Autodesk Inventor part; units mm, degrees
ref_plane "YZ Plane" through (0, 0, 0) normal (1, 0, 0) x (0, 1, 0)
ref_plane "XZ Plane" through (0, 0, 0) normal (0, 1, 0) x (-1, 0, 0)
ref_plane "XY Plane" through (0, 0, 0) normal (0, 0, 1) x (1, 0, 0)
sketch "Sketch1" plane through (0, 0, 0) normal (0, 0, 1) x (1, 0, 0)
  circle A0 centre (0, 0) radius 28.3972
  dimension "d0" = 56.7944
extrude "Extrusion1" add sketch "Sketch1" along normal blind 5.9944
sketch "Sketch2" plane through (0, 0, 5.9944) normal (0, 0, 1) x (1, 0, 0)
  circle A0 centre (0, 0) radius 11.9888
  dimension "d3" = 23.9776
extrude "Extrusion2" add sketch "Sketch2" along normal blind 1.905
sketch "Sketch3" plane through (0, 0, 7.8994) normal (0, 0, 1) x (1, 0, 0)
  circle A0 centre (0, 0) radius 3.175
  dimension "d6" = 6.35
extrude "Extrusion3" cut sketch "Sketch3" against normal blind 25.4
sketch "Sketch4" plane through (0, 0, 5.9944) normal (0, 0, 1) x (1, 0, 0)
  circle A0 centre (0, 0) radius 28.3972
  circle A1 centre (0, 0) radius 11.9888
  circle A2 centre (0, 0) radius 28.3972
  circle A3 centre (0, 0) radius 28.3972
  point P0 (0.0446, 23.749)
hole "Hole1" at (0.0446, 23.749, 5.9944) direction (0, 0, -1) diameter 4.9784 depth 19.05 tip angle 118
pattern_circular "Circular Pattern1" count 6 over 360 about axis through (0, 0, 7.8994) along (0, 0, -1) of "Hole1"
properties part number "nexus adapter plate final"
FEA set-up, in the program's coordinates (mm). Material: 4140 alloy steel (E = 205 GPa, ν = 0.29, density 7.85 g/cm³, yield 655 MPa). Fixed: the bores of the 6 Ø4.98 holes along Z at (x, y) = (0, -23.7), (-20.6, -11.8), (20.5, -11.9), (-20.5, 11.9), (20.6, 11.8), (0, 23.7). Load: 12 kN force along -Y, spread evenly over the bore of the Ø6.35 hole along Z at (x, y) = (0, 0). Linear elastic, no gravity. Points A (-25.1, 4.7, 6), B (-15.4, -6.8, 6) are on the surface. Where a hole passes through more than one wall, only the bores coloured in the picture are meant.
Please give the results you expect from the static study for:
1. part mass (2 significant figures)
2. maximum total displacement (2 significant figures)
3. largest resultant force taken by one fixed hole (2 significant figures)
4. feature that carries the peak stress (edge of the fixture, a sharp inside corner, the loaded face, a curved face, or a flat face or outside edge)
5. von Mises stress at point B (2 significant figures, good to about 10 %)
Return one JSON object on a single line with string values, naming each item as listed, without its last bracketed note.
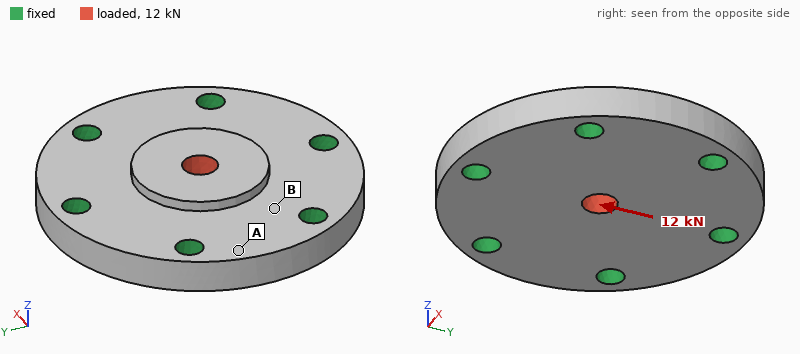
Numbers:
{"part mass": "120 g", "maximum total displacement": "5.2 µm", "largest resultant force taken by one fixed hole": "3.1 kN", "feature that carries the peak stress": "the loaded face", "von Mises stress at point B": "28 MPa"}
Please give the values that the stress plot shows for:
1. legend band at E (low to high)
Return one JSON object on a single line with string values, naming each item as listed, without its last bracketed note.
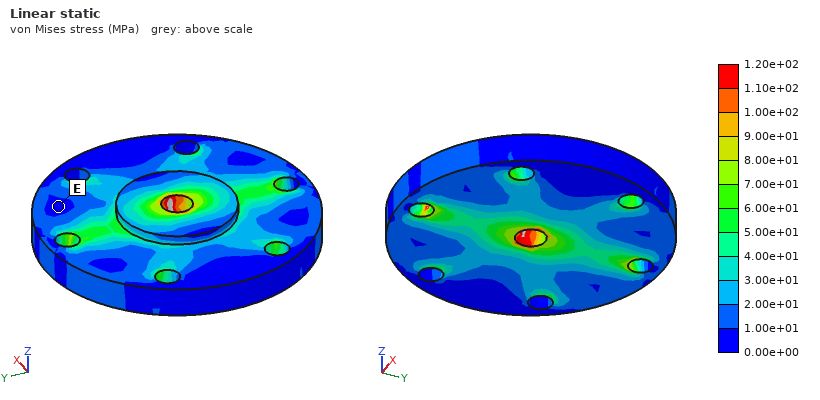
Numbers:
{"legend band at E": "0.00e+00 to 1.00e+01 MPa"}
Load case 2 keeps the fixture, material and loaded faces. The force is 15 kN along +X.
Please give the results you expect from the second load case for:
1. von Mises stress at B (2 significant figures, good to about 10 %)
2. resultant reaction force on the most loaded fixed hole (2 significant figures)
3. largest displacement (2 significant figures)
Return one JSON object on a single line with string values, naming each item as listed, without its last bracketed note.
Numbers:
{"von Mises stress at B": "57 MPa", "resultant reaction force on the most loaded fixed hole": "3.4 kN", "largest displacement": "6.6 µm"}
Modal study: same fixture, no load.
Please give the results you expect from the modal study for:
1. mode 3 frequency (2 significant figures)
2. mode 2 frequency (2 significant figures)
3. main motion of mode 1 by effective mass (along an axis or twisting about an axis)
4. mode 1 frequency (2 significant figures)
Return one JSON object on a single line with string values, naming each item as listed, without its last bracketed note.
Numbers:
{"mode 3 frequency": "39 kHz", "mode 2 frequency": "39 kHz", "main motion of mode 1 by effective mass": "along Z", "mode 1 frequency": "22 kHz"}
